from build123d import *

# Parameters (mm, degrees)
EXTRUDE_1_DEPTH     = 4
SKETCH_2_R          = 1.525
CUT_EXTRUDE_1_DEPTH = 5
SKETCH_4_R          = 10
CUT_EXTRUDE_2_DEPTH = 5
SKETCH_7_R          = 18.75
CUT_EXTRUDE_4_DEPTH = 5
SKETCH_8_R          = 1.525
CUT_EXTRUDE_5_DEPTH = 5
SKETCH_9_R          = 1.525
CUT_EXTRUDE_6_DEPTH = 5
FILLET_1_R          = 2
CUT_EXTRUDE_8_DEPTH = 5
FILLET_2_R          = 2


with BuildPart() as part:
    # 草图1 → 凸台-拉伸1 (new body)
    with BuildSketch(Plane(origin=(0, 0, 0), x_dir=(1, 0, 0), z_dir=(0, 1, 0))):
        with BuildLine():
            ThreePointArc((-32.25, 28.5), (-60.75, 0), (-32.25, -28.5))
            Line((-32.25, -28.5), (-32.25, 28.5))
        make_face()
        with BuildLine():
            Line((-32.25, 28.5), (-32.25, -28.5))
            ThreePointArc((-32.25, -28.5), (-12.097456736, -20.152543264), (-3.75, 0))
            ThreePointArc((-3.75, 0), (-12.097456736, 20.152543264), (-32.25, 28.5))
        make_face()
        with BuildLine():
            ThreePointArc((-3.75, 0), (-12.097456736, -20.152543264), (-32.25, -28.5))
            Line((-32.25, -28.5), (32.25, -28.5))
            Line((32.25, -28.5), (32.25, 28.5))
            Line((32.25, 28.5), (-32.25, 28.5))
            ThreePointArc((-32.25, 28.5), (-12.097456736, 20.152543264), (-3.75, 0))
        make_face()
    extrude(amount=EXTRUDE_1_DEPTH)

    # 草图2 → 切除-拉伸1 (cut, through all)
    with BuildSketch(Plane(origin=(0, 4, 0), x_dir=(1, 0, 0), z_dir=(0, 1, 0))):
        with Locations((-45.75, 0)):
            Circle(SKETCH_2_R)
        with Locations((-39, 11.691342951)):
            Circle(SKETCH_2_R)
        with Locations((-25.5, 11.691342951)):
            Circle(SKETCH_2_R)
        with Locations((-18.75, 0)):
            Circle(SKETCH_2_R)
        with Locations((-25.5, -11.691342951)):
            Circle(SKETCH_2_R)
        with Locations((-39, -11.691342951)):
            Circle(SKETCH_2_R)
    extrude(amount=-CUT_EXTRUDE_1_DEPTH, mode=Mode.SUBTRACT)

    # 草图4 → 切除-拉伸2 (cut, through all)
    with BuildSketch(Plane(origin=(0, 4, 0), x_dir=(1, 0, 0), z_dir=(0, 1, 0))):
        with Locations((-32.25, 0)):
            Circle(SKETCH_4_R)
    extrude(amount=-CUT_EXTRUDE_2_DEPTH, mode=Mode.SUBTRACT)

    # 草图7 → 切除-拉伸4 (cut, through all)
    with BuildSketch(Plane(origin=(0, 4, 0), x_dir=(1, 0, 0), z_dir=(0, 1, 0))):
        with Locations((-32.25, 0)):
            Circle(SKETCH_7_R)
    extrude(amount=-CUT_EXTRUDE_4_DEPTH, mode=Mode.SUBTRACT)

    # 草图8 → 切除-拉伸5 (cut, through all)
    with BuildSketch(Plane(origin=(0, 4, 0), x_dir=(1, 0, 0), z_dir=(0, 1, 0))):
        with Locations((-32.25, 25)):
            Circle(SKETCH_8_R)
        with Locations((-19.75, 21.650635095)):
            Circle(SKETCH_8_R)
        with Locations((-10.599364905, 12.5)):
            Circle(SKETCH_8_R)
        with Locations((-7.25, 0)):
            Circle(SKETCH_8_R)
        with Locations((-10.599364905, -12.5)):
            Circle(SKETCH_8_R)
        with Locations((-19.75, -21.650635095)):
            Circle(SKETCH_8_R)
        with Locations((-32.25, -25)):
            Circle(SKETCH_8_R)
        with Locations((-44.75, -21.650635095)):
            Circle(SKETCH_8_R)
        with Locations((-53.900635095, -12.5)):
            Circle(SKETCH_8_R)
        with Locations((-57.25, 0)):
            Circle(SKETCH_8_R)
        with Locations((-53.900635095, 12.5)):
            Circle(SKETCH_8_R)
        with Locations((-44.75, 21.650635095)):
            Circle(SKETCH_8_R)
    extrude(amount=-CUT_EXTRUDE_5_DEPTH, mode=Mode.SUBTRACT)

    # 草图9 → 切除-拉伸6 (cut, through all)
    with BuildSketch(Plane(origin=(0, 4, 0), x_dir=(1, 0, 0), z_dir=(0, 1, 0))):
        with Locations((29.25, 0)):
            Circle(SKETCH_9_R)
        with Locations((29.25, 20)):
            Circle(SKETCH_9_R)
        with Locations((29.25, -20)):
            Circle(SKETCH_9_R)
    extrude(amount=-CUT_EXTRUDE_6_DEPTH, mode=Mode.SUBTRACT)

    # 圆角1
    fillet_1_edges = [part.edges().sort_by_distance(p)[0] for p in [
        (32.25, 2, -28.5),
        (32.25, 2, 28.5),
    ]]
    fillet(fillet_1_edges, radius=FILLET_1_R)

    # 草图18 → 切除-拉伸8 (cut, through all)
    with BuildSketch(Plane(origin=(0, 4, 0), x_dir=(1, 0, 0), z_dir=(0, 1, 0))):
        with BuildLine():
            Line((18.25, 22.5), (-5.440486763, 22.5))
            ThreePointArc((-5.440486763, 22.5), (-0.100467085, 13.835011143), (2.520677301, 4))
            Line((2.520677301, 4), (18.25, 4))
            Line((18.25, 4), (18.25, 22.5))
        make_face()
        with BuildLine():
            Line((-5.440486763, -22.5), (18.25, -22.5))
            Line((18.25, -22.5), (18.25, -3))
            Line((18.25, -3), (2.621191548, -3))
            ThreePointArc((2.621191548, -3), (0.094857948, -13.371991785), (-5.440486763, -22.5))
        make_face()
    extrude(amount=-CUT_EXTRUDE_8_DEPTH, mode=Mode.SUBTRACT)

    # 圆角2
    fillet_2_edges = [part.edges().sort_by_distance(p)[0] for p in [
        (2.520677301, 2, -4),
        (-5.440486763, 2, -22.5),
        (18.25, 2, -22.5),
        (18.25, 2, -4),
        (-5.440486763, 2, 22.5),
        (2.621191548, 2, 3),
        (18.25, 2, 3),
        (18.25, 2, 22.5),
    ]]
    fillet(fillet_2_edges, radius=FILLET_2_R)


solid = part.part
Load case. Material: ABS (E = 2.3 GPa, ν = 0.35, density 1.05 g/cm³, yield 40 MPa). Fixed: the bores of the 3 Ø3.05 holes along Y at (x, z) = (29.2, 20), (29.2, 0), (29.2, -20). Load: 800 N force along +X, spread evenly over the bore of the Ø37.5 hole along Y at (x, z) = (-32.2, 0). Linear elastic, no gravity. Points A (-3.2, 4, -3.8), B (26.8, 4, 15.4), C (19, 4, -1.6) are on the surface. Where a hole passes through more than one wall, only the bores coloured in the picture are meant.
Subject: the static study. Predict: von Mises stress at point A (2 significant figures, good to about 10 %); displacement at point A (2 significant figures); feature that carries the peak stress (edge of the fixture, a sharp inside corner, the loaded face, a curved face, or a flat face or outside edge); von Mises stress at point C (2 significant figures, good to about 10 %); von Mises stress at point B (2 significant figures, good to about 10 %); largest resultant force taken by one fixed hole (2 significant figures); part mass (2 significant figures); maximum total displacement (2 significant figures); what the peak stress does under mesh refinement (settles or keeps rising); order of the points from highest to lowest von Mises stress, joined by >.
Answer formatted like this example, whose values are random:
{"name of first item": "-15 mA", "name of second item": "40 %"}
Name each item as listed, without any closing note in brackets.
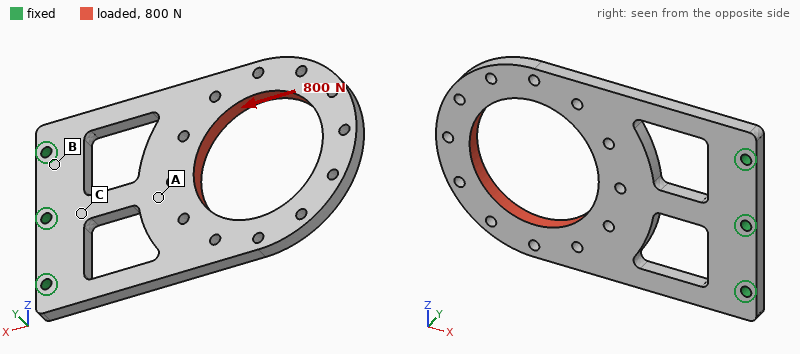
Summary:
{"von Mises stress at point A": "6.0 MPa", "displacement at point A": "0.12 mm", "feature that carries the peak stress": "edge of the fixture", "von Mises stress at point C": "8.3 MPa", "von Mises stress at point B": "2.5 MPa", "largest resultant force taken by one fixed hole": "310 N", "part mass": "13 g", "maximum total displacement": "0.47 mm", "what the peak stress does under mesh refinement": "keeps rising", "order of the points from highest to lowest von Mises stress, joined by >": "C > A > B"}
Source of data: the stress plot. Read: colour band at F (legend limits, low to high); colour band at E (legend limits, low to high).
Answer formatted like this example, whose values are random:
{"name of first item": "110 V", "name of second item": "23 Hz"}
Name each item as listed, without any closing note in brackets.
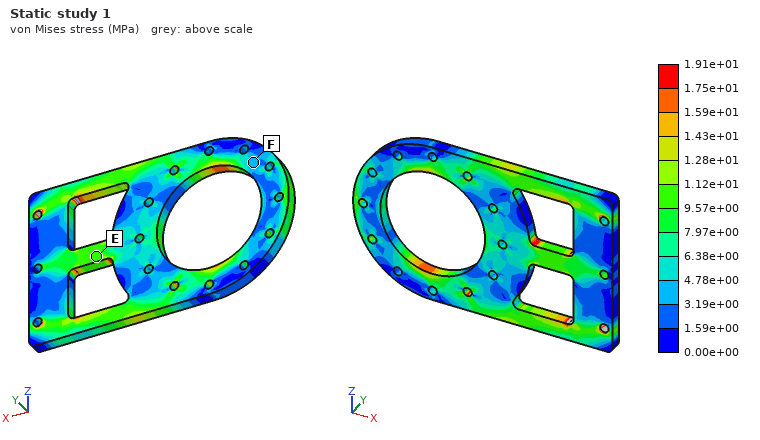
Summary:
{"colour band at F": "3.19e+00 to 4.78e+00 MPa", "colour band at E": "9.57e+00 to 1.12e+01 MPa"}
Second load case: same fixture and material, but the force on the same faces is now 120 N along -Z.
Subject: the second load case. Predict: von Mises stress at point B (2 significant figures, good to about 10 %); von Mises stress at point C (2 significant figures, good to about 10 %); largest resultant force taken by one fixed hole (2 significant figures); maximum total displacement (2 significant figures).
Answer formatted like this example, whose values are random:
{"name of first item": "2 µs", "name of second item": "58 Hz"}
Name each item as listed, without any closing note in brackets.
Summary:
{"von Mises stress at point B": "3.5 MPa", "von Mises stress at point C": "3.4 MPa", "largest resultant force taken by one fixed hole": "170 N", "maximum total displacement": "0.68 mm"}
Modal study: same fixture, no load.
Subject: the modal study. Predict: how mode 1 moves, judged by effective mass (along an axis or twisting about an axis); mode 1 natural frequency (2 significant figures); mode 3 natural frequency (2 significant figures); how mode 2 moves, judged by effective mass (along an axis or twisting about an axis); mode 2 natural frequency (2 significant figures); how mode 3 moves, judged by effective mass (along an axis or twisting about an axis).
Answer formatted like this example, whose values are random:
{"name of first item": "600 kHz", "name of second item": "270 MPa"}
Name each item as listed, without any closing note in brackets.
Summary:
{"how mode 1 moves, judged by effective mass": "along Y", "mode 1 natural frequency": "120 Hz", "mode 3 natural frequency": "630 Hz", "how mode 2 moves, judged by effective mass": "twisting about X", "mode 2 natural frequency": "380 Hz", "how mode 3 moves, judged by effective mass": "along Y"}
